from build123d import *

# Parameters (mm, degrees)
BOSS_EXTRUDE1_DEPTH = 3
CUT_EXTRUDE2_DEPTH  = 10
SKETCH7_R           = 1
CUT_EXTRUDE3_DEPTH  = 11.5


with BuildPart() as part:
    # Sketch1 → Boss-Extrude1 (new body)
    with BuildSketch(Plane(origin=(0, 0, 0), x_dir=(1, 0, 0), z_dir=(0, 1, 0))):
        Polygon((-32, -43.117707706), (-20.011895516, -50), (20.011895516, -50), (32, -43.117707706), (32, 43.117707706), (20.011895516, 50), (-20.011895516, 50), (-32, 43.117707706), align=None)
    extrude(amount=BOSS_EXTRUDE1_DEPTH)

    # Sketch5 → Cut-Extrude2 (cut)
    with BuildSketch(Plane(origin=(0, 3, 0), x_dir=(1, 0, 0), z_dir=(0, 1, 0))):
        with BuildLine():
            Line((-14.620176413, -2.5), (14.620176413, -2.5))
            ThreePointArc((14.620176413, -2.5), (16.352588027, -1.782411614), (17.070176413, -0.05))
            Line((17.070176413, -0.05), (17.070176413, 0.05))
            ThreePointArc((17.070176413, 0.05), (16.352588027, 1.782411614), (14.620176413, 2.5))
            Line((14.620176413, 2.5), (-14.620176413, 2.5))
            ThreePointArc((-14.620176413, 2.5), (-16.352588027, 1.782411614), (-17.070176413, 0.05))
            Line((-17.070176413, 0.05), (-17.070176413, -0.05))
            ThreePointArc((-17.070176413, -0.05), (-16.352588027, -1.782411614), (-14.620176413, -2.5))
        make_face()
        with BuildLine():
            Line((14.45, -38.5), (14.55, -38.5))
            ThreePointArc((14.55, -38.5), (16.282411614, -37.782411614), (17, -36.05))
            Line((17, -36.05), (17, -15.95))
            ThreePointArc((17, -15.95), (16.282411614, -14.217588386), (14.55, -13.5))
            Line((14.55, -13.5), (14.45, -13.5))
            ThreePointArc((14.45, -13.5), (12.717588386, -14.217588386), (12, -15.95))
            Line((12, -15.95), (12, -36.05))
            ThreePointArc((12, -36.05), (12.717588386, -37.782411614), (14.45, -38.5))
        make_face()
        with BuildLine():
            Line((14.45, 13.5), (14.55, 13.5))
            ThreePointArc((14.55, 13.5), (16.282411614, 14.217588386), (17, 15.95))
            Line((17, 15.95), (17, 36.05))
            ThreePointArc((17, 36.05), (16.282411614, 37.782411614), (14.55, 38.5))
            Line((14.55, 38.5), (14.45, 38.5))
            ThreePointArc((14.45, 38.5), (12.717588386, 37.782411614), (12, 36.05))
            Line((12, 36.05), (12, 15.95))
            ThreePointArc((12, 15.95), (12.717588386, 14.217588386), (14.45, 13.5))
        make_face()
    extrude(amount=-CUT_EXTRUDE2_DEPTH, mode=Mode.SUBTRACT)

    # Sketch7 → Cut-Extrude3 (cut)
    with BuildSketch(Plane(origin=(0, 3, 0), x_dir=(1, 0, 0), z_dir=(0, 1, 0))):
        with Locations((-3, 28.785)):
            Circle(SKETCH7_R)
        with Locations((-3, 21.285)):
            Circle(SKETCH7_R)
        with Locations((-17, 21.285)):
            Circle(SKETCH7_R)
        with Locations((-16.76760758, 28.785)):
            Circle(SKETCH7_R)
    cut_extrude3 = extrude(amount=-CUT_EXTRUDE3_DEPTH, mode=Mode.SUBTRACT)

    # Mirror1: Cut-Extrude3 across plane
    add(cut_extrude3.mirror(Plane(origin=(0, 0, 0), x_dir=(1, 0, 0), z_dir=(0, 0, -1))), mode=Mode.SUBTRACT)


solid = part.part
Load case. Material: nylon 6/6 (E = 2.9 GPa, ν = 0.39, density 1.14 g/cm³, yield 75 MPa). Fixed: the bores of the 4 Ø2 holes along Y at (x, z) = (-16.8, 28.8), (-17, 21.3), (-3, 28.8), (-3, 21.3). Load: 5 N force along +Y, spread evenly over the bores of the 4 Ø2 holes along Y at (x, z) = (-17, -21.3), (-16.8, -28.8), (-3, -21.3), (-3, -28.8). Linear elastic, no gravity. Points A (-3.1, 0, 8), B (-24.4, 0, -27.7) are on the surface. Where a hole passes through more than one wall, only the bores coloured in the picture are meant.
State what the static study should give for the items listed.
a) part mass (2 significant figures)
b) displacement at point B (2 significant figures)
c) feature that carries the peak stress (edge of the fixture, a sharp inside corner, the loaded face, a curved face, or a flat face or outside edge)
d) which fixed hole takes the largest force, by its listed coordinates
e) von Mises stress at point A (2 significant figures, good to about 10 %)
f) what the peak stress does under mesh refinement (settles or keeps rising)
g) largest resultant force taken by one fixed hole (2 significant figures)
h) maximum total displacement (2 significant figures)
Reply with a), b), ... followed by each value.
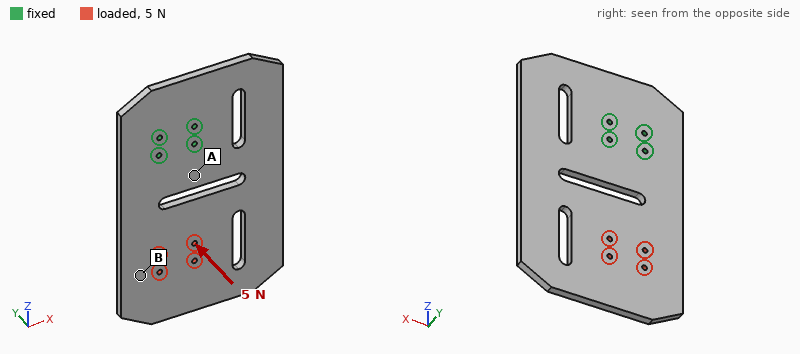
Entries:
a) 20 g
b) 0.73 mm
c) edge of the fixture
d) (-3, 21.3)
e) 1.2 MPa
f) keeps rising
g) 11 N
h) 1.2 mm
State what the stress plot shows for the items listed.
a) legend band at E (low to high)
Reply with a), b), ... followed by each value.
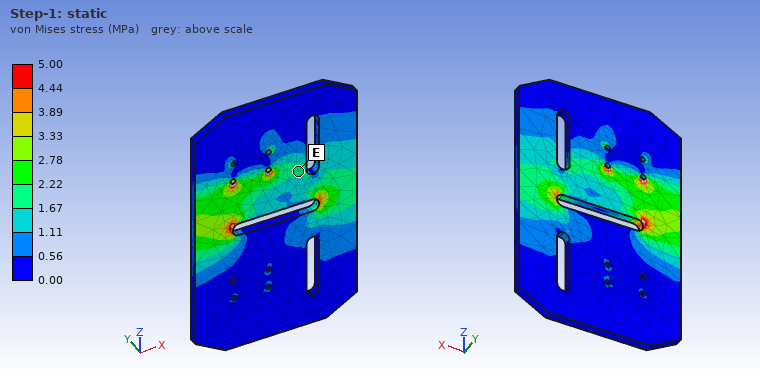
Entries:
a) 1.67 to 2.22 MPa
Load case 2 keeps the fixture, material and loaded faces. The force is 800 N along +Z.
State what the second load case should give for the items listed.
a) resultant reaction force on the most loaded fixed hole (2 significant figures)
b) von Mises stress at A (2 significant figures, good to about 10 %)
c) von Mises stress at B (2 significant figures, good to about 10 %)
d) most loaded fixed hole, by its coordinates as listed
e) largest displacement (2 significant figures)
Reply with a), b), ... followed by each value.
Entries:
a) 280 N
b) 4.0 MPa
c) 5.2 MPa
d) (-17, 21.3)
e) 0.27 mm
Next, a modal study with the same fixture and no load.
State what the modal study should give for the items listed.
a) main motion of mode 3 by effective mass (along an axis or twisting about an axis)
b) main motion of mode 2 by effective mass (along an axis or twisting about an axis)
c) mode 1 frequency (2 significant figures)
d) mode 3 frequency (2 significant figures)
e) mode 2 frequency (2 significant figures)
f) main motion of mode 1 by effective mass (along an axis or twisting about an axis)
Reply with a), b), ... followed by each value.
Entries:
a) along Y
b) twisting about Z
c) 120 Hz
d) 600 Hz
e) 310 Hz
f) along Y
